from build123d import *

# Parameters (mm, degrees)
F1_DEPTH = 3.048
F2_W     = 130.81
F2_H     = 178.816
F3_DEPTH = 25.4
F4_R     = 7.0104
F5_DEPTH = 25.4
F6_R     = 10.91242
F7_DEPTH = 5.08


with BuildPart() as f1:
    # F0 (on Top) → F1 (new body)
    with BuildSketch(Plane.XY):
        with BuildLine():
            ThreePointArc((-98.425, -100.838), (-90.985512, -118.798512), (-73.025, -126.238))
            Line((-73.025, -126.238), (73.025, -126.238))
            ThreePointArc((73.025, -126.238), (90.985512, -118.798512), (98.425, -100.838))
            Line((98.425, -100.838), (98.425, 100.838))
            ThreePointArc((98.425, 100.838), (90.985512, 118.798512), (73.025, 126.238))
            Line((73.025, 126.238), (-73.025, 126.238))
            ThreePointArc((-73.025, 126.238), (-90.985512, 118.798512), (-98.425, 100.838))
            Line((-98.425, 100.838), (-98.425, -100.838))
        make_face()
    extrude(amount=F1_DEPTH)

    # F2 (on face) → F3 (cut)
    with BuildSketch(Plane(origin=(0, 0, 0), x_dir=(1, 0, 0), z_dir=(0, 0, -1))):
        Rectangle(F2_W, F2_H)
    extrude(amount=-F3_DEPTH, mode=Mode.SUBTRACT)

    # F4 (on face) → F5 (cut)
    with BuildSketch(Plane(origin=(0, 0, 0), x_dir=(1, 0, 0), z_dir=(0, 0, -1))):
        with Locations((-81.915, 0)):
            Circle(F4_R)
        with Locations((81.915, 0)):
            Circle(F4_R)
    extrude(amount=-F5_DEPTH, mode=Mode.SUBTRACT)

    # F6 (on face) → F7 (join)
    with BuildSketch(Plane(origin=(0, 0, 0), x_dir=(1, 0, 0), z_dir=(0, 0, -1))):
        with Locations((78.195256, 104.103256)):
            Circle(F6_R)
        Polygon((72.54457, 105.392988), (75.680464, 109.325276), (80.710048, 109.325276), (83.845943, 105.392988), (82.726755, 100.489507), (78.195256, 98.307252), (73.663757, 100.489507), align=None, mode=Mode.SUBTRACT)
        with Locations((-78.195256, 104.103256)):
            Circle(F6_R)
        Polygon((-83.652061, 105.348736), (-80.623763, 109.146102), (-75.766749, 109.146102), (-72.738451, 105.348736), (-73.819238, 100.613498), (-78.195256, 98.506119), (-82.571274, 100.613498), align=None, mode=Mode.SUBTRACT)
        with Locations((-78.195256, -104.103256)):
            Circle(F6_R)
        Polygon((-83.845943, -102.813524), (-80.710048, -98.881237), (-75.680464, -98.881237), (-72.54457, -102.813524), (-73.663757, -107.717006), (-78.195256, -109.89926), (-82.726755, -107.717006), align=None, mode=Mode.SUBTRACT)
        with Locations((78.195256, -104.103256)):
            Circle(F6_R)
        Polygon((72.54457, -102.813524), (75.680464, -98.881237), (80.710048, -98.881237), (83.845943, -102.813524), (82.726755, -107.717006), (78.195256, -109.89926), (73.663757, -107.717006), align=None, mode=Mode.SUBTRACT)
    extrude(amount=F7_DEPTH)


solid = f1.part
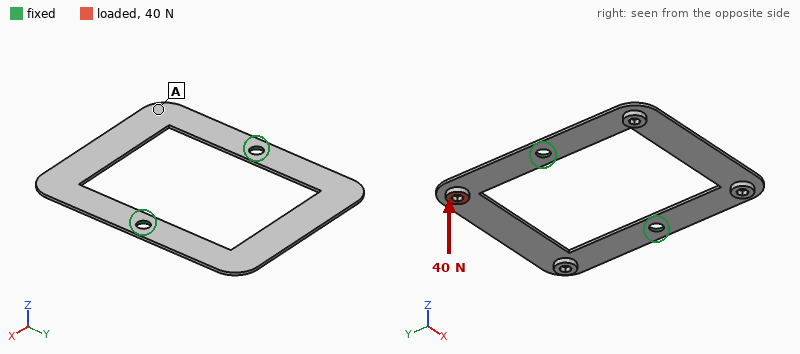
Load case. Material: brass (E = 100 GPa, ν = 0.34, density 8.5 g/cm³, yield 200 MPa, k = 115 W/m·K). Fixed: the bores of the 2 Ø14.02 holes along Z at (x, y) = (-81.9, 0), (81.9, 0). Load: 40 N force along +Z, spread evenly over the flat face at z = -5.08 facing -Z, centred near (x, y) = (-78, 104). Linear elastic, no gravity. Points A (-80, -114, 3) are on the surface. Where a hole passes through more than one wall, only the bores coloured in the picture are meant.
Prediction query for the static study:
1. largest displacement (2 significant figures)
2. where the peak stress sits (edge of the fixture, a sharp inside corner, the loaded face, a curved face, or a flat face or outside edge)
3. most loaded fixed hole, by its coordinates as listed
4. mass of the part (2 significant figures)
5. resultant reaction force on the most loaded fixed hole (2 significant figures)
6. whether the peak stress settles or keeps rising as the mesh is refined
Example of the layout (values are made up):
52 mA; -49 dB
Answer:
1.4 mm; edge of the fixture; (-81.9, 0); 710 g; 35 N; keeps rising
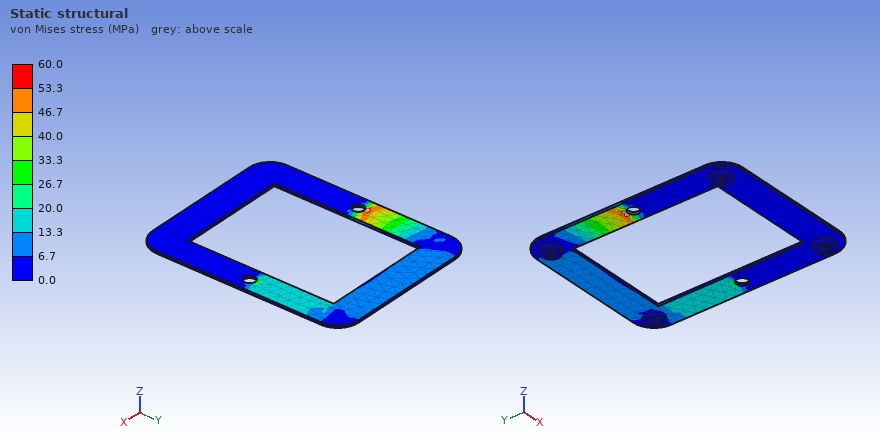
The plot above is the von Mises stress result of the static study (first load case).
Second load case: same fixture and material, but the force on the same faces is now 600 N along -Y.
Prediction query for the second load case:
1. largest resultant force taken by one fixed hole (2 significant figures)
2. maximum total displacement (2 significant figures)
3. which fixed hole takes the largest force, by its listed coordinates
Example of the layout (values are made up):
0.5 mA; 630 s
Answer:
590 N; 2.1 mm; (-81.9, 0)
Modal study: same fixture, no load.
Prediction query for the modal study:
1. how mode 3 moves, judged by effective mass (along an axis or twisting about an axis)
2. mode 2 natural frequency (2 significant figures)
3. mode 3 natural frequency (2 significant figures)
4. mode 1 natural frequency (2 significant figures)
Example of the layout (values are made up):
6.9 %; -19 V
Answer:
twisting about Y; 70 Hz; 160 Hz; 70 Hz
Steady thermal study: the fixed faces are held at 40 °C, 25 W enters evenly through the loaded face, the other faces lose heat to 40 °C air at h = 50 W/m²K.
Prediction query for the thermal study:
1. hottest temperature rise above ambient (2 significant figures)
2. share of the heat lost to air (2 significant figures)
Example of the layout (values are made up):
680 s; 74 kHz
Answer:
55 K; 84 %
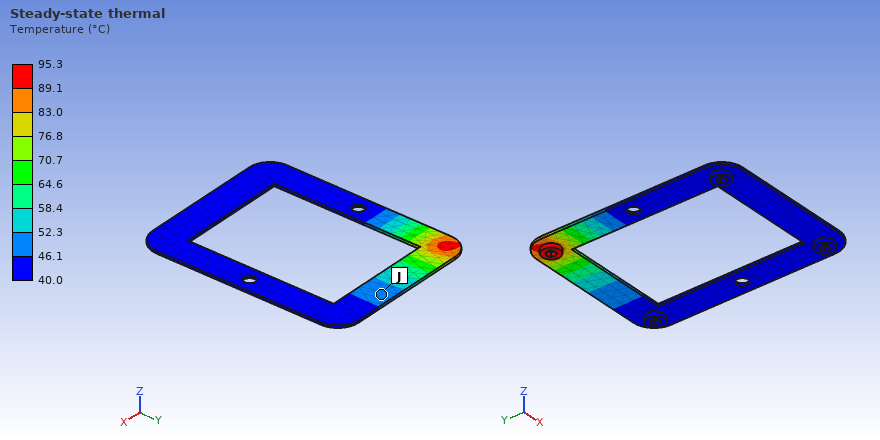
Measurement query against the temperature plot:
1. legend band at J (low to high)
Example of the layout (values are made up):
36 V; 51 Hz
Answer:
46.1 to 52.3 °C
